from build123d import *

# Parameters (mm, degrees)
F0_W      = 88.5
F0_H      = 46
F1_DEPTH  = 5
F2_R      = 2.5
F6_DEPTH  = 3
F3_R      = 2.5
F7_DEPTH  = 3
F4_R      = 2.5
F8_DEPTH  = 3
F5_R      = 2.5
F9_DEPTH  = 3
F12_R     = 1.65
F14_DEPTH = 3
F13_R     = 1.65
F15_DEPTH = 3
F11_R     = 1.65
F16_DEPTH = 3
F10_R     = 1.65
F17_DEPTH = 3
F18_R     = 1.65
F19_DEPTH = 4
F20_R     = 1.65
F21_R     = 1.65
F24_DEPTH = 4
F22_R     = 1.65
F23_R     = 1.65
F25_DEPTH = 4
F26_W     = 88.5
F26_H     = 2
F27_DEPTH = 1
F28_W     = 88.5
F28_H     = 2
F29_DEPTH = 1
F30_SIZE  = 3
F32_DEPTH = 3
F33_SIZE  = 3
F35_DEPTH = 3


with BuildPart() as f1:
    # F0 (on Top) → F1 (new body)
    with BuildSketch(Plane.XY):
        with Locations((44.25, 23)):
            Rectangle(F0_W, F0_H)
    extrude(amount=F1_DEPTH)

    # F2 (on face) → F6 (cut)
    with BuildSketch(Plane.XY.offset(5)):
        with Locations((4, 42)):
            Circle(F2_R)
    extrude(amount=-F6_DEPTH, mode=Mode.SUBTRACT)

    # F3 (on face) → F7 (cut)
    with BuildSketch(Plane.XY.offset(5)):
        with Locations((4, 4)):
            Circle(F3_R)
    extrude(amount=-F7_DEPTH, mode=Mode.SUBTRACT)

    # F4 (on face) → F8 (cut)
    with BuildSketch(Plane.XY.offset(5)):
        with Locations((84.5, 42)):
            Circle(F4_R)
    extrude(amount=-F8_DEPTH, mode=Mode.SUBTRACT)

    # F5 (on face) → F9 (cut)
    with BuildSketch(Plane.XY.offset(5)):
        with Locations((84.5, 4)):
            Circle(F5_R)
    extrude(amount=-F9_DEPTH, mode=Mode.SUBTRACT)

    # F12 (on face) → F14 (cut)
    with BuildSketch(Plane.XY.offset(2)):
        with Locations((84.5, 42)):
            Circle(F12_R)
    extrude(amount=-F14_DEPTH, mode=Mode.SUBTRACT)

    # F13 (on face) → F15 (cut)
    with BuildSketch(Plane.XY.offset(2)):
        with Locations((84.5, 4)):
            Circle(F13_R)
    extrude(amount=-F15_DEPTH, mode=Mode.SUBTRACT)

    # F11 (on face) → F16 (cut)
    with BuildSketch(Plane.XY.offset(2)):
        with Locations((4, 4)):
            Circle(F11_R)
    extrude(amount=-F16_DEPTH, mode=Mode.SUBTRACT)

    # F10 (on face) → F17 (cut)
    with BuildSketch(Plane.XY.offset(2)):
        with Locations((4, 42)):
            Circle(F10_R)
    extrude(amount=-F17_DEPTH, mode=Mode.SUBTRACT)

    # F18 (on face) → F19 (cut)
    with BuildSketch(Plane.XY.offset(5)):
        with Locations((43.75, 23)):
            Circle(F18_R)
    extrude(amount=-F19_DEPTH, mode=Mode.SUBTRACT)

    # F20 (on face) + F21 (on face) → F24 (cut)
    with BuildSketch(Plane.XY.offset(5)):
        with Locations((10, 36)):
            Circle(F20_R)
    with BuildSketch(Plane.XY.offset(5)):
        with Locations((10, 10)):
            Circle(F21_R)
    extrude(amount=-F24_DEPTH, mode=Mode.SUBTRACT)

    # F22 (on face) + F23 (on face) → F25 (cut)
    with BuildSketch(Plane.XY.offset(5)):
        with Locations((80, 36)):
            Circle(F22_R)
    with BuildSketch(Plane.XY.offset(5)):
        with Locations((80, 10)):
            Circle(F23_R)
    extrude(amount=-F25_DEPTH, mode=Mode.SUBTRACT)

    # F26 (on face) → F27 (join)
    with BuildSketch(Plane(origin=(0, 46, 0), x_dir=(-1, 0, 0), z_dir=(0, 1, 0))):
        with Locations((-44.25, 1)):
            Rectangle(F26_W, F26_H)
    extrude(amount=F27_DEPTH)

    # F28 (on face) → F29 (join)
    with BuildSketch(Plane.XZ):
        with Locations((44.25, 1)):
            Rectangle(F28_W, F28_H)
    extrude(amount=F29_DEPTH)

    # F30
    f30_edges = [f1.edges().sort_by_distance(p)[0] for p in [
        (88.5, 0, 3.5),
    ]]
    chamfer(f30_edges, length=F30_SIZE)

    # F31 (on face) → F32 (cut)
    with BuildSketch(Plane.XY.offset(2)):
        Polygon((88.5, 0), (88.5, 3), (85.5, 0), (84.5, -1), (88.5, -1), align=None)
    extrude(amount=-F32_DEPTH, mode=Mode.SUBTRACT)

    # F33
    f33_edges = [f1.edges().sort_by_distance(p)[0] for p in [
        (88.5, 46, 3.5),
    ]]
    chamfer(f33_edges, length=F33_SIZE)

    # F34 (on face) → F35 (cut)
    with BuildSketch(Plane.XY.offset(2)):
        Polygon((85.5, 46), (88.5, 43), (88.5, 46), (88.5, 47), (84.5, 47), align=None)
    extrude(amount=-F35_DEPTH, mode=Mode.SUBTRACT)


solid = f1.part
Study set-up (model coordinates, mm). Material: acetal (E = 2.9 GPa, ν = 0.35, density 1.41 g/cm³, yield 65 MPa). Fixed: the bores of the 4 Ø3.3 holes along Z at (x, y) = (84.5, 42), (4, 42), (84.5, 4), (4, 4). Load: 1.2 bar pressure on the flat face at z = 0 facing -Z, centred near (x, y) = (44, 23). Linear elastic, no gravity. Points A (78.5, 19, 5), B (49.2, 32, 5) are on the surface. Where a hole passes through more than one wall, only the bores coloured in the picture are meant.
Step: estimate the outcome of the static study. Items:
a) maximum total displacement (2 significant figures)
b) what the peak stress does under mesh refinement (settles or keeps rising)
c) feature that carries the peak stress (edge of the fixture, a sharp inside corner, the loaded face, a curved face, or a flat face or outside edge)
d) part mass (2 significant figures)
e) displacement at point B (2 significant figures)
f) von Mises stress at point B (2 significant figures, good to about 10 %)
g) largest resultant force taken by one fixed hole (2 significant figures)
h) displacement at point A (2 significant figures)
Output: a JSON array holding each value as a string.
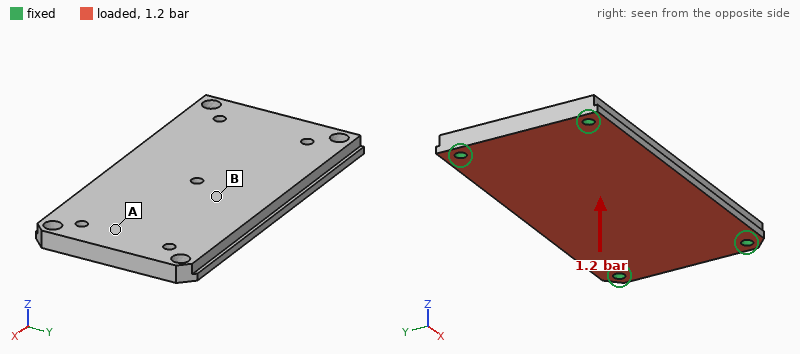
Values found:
["0.98 mm", "keeps rising", "edge of the fixture", "28 g", "0.90 mm", "13 MPa", "240 N", "0.24 mm"]
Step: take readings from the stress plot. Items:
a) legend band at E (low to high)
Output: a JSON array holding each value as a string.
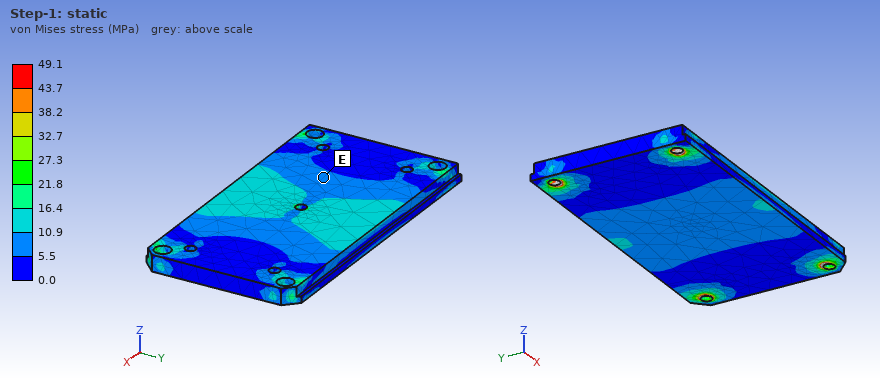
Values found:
["5.5 to 10.9 MPa"]
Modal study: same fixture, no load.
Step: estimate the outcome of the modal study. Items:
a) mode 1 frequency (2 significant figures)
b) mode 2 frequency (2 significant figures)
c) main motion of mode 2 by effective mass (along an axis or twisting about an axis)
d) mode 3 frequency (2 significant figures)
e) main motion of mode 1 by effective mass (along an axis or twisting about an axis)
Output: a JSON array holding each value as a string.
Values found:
["780 Hz", "1400 Hz", "twisting about X", "2200 Hz", "along Z"]
